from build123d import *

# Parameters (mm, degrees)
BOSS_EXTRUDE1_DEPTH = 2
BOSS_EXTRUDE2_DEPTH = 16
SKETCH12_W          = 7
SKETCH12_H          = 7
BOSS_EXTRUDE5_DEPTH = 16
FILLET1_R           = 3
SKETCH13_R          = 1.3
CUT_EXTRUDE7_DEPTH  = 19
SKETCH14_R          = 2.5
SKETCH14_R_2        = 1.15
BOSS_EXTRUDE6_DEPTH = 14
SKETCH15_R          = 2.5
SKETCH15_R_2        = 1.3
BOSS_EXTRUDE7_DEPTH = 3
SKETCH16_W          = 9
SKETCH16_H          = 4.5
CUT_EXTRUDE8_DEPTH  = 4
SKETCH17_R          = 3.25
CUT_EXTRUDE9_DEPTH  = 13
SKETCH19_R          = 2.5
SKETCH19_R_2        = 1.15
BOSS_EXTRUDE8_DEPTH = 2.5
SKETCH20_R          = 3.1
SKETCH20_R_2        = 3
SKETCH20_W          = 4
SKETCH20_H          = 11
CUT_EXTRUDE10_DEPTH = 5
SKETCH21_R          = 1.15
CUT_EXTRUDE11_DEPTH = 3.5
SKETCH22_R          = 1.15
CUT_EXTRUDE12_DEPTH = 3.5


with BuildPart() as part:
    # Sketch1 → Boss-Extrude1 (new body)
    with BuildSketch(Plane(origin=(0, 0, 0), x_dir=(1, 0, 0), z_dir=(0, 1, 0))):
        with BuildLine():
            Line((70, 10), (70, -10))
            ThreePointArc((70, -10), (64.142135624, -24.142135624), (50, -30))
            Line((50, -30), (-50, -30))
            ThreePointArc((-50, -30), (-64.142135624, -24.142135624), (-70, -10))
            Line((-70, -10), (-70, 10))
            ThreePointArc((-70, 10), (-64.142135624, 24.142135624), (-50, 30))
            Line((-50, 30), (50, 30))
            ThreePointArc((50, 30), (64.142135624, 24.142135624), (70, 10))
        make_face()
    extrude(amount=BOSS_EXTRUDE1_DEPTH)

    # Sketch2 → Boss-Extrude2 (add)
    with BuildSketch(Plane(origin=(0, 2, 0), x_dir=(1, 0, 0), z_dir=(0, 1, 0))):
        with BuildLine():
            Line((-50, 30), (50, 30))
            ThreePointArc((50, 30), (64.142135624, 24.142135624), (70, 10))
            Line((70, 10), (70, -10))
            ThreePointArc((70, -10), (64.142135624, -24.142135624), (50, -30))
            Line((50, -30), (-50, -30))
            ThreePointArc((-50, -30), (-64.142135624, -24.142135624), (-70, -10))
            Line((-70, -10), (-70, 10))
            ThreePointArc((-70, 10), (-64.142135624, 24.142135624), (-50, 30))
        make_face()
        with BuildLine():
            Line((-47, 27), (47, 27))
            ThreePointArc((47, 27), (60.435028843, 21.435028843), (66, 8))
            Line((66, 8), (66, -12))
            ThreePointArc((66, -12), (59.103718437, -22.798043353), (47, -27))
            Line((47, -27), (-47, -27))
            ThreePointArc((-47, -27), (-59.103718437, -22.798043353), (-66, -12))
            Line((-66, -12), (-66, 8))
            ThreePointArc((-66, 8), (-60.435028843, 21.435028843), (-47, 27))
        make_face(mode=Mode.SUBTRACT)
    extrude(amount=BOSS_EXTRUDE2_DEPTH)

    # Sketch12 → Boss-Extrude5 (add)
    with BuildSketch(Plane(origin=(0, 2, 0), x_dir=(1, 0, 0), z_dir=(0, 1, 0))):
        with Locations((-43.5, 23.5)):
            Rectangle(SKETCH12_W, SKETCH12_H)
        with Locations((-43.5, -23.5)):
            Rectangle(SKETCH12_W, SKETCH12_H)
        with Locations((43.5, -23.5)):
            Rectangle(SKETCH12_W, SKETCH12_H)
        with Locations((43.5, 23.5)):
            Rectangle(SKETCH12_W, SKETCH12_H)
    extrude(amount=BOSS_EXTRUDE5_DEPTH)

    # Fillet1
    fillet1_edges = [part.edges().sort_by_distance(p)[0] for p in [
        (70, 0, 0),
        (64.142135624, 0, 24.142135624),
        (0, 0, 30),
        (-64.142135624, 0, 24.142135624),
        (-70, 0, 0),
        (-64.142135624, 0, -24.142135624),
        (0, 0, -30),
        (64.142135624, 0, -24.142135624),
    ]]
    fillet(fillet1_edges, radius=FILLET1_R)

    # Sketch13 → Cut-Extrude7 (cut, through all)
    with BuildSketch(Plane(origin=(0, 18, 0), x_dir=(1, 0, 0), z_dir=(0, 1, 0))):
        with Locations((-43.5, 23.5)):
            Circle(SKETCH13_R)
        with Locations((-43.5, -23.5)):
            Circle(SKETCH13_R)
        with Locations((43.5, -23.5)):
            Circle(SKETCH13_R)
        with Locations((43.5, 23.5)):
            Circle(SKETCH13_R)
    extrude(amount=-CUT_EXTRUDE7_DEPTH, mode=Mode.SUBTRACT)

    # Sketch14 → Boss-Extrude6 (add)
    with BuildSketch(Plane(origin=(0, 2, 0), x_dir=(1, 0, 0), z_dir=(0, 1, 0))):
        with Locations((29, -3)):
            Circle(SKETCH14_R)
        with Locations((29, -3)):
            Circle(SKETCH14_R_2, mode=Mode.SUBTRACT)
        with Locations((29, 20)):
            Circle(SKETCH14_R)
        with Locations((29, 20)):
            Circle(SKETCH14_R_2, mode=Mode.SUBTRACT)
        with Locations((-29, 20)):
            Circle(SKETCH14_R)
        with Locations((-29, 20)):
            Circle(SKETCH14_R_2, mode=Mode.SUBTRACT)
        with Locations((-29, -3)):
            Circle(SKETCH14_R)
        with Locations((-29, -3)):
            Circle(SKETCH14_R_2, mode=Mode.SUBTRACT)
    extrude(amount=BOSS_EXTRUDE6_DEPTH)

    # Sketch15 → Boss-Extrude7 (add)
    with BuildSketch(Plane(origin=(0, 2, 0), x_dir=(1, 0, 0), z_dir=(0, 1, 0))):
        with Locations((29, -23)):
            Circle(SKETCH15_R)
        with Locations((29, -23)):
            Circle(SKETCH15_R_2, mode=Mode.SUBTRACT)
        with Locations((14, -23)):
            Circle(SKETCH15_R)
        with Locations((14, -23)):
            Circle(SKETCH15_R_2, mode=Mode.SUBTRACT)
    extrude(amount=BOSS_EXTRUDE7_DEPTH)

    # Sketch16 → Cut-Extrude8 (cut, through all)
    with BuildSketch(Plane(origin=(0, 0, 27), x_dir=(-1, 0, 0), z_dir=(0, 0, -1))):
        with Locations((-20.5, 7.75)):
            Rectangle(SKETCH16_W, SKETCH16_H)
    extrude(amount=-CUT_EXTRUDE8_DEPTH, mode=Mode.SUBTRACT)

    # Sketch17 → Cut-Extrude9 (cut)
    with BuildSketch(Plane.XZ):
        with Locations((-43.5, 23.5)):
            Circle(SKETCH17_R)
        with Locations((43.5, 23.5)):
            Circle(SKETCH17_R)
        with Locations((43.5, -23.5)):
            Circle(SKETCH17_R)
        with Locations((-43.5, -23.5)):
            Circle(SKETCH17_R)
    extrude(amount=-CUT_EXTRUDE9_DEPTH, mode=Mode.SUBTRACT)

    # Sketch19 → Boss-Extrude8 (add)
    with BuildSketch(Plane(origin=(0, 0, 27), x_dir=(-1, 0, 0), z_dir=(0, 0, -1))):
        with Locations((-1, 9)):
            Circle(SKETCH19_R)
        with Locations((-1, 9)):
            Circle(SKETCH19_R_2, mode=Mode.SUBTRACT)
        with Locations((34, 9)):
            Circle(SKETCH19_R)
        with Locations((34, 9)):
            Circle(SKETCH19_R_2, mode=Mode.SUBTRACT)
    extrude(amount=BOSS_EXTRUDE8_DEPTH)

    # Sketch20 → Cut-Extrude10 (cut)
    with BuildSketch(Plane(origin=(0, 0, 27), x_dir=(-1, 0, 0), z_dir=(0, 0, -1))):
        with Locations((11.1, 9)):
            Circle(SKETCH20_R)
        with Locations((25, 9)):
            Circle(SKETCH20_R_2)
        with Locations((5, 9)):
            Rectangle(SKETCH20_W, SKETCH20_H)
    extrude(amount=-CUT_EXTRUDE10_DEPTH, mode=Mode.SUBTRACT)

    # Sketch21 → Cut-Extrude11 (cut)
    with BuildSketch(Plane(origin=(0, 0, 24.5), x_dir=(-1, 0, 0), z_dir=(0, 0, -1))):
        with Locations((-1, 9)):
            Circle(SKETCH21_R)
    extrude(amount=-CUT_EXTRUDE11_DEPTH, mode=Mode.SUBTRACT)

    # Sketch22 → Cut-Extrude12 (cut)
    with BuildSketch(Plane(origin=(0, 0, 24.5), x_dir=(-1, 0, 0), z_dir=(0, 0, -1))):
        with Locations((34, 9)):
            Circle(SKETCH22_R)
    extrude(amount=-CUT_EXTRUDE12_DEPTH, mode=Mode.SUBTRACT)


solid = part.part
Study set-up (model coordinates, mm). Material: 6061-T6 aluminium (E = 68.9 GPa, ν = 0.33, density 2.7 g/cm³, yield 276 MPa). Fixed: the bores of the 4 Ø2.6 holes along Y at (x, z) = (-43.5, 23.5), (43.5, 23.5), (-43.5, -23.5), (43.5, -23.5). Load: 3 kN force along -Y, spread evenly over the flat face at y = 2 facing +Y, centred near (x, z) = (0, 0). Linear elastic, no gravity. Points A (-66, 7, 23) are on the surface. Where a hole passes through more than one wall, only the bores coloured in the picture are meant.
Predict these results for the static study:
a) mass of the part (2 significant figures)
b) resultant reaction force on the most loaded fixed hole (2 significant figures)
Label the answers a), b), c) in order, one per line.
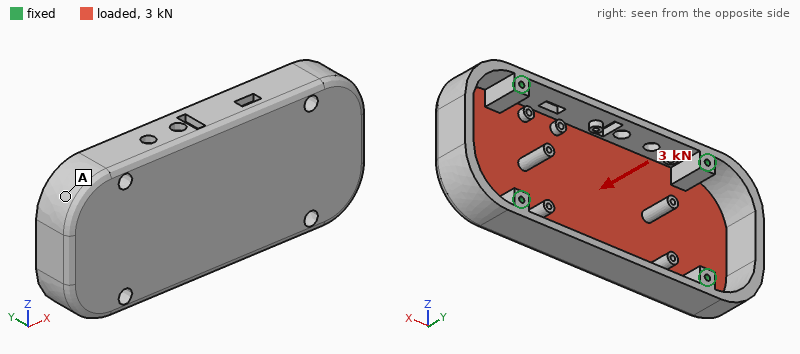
a) 100 g
b) 820 N
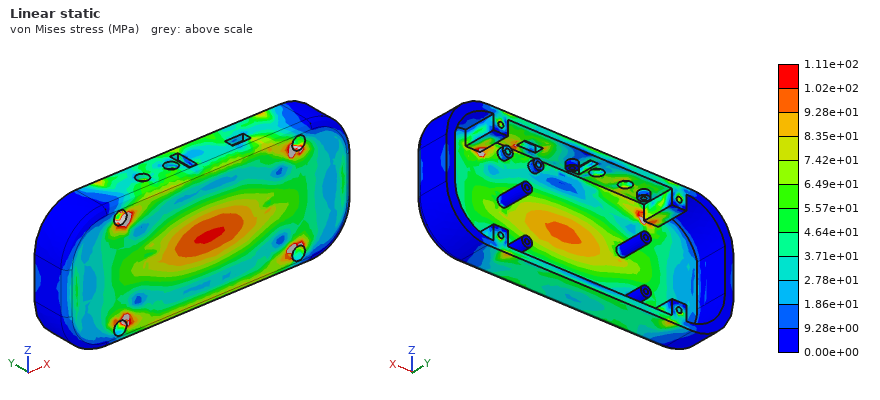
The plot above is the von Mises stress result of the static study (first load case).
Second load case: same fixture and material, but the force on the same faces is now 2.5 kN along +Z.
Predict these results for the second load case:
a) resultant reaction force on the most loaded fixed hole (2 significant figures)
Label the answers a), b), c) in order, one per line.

a) 650 N
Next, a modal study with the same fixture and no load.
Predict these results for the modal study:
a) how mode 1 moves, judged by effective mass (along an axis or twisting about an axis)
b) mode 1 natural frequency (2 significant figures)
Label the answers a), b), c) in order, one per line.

a) along Y
b) 2600 Hz
